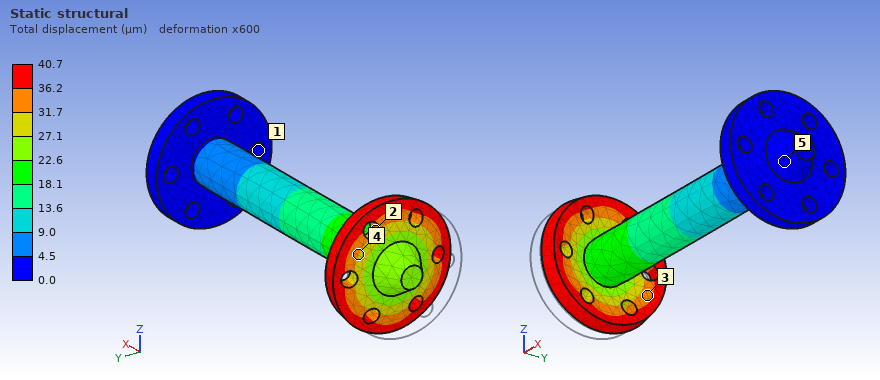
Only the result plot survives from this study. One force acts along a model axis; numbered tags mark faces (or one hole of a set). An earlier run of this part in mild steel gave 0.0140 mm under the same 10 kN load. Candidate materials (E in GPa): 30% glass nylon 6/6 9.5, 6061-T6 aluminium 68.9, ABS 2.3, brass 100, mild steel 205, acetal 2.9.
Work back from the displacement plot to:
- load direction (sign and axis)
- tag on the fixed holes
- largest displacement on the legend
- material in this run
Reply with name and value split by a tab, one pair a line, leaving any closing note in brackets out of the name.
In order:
load direction	+X
tag on the fixed holes	1
largest displacement on the legend	40.7 µm
material in this run	6061-T6 aluminium
